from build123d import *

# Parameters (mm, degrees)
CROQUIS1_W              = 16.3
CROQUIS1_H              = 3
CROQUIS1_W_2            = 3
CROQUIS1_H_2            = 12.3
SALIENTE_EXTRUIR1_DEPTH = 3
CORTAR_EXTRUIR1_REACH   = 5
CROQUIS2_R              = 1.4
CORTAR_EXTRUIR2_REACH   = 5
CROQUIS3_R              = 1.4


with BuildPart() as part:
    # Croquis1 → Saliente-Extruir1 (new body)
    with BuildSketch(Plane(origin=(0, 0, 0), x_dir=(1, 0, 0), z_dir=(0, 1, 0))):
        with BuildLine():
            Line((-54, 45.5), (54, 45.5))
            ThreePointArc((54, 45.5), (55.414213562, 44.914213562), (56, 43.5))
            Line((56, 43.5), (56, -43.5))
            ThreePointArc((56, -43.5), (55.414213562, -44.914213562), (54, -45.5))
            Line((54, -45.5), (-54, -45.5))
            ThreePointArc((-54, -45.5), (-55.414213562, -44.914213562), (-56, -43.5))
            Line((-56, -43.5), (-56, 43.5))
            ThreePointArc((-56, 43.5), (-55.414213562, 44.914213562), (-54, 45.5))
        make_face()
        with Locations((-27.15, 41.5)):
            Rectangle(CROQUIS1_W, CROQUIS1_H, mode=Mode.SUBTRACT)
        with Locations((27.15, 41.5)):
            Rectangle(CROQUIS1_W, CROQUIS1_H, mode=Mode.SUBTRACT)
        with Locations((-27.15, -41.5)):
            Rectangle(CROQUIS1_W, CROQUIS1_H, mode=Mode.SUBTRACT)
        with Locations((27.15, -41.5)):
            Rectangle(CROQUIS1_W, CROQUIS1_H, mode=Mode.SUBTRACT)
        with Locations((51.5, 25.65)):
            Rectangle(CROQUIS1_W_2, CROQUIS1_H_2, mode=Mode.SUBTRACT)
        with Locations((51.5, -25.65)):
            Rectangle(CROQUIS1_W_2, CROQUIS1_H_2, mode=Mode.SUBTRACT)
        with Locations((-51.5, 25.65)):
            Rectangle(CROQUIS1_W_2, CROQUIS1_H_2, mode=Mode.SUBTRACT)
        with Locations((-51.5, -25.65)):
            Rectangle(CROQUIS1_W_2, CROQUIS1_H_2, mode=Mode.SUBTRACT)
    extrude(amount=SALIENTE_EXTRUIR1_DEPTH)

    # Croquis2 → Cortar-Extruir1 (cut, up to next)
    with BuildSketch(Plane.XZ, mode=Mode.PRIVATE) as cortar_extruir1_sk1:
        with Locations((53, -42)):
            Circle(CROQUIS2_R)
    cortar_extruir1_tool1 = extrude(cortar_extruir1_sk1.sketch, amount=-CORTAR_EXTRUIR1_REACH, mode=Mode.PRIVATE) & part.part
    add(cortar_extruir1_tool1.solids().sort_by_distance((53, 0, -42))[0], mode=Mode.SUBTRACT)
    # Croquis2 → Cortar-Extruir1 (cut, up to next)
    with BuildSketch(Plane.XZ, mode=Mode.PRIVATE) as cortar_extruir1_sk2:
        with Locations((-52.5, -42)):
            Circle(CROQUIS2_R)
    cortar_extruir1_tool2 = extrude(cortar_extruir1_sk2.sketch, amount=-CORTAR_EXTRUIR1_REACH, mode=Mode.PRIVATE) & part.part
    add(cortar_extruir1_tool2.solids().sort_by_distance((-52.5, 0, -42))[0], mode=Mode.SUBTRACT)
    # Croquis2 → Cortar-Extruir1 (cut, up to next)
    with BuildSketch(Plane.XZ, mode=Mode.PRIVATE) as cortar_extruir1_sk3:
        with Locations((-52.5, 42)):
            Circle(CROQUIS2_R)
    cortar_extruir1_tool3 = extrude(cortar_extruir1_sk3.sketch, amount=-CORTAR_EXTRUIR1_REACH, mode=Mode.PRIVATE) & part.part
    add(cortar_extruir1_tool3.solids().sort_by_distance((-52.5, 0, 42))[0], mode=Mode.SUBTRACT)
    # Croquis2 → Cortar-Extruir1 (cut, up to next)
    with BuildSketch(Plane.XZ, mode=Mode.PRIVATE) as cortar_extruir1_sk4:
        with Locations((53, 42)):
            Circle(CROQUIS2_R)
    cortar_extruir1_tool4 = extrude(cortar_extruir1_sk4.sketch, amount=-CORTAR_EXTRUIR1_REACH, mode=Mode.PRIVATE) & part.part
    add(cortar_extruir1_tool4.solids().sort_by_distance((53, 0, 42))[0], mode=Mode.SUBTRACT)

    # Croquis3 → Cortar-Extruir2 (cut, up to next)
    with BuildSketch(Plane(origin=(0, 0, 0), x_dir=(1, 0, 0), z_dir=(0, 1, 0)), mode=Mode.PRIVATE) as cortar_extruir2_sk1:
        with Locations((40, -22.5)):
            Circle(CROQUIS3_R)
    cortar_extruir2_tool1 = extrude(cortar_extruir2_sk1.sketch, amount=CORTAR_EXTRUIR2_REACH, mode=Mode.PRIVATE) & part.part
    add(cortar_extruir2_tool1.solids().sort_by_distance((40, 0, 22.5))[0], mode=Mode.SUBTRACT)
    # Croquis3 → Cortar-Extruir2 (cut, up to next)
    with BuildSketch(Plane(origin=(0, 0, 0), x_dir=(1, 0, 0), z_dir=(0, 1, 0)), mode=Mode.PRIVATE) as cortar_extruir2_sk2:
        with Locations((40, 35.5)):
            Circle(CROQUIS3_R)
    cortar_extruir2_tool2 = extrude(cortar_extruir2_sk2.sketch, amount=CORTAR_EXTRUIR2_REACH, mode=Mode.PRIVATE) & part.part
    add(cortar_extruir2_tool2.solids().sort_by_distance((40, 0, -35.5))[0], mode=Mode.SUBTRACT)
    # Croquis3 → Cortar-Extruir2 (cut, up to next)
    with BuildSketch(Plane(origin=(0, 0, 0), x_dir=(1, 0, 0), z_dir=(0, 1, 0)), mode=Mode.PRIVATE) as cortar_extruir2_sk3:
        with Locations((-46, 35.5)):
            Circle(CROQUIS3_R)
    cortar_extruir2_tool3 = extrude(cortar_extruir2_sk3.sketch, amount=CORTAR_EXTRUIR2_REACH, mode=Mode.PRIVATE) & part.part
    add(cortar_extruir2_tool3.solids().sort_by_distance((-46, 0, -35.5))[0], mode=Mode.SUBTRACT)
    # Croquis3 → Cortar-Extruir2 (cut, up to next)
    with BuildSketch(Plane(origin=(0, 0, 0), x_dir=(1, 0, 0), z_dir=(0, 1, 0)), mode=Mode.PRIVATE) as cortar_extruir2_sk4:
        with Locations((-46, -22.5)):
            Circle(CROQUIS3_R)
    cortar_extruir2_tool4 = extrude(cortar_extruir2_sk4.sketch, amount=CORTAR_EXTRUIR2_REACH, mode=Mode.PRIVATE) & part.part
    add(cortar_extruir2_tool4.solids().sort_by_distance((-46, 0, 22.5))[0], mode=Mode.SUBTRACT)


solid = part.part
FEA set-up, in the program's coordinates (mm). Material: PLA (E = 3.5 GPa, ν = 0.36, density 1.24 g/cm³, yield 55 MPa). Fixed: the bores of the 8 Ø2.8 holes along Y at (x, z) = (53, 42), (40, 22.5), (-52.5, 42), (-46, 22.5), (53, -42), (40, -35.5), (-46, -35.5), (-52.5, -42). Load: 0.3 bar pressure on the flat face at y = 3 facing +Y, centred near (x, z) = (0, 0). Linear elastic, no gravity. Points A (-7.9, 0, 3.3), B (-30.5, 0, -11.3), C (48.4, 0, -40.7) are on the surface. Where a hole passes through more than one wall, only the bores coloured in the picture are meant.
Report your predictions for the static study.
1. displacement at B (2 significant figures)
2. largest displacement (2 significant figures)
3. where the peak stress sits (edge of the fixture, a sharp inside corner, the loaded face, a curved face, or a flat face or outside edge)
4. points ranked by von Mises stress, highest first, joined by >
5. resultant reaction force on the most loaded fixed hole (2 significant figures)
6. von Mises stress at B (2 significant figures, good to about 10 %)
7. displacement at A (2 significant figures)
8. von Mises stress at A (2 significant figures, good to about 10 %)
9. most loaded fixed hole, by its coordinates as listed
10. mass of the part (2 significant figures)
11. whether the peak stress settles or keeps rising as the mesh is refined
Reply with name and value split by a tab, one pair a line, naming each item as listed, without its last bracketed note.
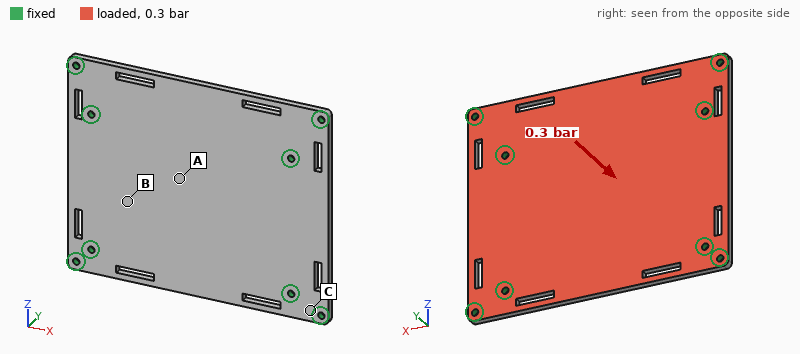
displacement at B	0.46 mm
largest displacement	0.82 mm
where the peak stress sits	edge of the fixture
points ranked by von Mises stress, highest first, joined by >	A > B > C
resultant reaction force on the most loaded fixed hole	93 N
von Mises stress at B	3.3 MPa
displacement at A	0.78 mm
von Mises stress at A	6.2 MPa
most loaded fixed hole, by its coordinates as listed	(40, 22.5)
mass of the part	36 g
whether the peak stress settles or keeps rising as the mesh is refined	keeps rising
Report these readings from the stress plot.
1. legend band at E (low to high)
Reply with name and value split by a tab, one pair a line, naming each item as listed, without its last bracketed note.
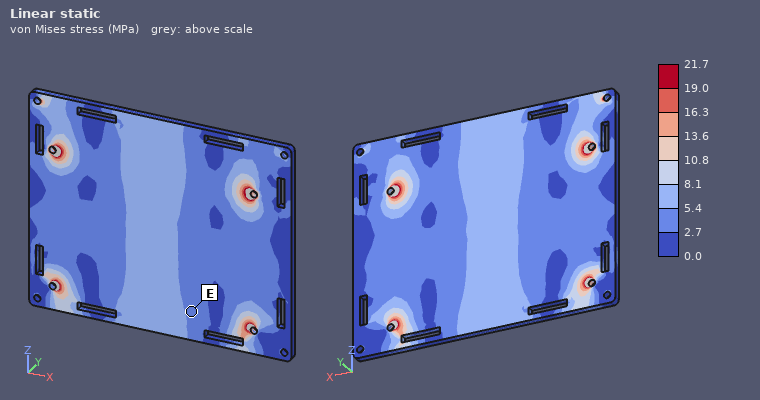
legend band at E	2.7 to 5.4 MPa
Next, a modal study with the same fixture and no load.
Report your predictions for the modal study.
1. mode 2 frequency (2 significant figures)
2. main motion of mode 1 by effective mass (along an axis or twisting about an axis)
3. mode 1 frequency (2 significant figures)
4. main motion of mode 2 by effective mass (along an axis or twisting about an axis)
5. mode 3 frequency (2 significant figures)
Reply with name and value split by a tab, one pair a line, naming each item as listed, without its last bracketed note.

mode 2 frequency	730 Hz
main motion of mode 1 by effective mass	along Y
mode 1 frequency	580 Hz
main motion of mode 2 by effective mass	twisting about X
mode 3 frequency	1100 Hz
